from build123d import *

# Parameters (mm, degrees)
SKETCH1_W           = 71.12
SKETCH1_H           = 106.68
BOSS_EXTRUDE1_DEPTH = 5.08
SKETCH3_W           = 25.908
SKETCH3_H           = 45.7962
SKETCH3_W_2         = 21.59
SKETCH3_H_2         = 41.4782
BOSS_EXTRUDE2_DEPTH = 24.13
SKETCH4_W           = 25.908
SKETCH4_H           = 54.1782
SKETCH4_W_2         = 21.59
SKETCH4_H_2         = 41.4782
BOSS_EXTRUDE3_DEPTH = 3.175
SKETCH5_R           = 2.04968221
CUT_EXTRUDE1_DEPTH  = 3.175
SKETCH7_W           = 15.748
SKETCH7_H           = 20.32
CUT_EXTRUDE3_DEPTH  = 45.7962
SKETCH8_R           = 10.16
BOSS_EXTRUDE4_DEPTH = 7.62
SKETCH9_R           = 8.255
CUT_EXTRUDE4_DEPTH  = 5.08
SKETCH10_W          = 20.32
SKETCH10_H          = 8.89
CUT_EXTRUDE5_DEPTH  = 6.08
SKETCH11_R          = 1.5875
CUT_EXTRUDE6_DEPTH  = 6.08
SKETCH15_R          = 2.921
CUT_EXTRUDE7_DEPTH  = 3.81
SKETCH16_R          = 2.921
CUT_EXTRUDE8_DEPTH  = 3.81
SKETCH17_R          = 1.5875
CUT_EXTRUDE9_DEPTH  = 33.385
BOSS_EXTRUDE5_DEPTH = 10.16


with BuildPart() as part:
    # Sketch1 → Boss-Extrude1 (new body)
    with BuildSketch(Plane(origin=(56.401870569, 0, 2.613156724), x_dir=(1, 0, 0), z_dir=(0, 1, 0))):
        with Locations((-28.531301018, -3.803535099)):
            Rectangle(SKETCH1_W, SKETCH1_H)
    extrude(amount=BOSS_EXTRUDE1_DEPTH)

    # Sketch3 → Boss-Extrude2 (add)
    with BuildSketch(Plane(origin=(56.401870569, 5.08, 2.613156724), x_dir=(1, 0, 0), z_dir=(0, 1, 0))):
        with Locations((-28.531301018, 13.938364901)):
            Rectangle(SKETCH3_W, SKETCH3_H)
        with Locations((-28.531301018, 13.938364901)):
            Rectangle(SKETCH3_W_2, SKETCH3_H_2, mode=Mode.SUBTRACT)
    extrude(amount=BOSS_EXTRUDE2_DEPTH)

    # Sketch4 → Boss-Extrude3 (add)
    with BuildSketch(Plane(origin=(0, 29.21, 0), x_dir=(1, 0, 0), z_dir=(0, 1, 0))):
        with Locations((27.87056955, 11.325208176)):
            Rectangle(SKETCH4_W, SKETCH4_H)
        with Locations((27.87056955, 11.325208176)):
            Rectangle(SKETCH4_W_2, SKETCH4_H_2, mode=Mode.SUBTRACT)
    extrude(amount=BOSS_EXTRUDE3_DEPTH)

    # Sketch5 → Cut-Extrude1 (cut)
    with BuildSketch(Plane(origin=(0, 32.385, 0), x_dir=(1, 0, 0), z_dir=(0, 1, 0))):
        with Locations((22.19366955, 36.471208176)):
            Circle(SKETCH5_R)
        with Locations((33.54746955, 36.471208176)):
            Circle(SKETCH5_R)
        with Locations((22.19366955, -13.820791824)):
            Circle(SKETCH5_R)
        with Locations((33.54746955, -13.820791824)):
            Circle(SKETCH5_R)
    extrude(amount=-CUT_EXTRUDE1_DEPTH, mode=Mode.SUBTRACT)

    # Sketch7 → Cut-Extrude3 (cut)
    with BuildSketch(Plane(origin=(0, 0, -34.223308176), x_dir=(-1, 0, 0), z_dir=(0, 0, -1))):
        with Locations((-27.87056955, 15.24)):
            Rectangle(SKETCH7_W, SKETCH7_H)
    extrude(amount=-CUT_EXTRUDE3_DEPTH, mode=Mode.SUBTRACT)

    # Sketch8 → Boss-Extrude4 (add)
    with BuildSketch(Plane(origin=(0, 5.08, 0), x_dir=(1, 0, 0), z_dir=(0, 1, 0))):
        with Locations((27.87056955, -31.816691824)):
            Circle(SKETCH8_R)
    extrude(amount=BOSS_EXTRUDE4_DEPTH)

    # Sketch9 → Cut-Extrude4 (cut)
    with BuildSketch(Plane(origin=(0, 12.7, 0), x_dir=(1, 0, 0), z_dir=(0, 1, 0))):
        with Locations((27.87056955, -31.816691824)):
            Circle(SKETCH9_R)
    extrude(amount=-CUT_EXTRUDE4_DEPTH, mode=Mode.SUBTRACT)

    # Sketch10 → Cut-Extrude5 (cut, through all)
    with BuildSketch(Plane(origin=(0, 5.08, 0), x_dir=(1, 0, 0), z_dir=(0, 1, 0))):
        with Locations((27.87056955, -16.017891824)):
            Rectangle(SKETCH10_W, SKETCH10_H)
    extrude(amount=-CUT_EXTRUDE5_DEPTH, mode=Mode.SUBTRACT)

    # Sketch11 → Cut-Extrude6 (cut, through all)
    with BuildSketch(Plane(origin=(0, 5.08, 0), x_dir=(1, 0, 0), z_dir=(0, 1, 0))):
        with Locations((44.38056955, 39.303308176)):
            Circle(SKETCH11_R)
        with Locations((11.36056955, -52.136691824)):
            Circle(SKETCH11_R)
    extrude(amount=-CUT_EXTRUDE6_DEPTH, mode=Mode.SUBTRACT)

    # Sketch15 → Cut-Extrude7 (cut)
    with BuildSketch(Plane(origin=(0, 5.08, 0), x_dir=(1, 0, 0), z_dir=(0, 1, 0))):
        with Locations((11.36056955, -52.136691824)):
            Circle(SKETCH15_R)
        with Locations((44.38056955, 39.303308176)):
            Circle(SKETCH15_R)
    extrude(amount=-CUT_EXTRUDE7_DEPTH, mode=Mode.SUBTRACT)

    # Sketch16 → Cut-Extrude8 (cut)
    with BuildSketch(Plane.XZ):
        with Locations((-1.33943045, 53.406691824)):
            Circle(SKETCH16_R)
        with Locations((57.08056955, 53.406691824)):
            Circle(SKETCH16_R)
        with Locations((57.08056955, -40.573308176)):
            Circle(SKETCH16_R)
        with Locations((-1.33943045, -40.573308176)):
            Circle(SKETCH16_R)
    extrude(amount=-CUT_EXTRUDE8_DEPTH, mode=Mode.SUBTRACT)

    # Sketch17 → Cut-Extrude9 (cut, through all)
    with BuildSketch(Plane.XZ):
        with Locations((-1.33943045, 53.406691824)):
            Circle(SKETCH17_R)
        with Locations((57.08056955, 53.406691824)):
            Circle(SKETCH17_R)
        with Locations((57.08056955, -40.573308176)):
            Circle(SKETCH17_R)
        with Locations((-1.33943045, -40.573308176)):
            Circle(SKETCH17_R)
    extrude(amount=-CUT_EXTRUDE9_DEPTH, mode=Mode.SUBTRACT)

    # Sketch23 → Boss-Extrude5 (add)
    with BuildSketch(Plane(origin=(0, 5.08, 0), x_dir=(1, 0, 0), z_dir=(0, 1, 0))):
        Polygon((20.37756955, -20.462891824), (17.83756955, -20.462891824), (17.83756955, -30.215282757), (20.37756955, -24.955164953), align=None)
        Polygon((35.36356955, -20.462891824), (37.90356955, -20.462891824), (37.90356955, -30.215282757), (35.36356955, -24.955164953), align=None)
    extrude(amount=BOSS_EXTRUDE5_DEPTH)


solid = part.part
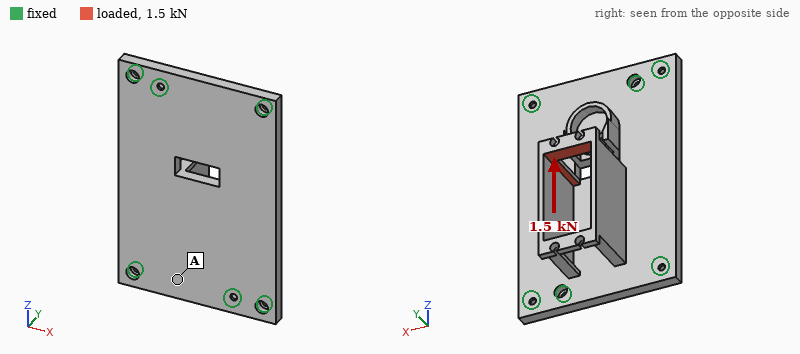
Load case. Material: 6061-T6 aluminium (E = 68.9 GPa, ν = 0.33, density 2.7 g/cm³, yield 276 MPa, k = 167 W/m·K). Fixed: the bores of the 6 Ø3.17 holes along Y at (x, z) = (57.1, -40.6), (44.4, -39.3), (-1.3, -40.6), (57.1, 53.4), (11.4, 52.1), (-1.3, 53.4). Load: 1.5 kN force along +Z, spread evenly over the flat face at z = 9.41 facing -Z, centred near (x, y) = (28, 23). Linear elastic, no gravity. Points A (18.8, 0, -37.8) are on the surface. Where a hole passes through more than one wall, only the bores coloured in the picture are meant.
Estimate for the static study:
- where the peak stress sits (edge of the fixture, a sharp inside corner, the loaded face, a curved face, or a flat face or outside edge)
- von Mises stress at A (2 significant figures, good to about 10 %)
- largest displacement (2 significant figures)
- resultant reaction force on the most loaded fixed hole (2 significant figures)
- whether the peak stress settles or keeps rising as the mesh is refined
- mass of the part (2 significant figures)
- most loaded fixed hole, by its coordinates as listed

a sharp inside corner
16 MPa
0.21 mm
970 N
keeps rising
120 g
(11.4, 52.1)
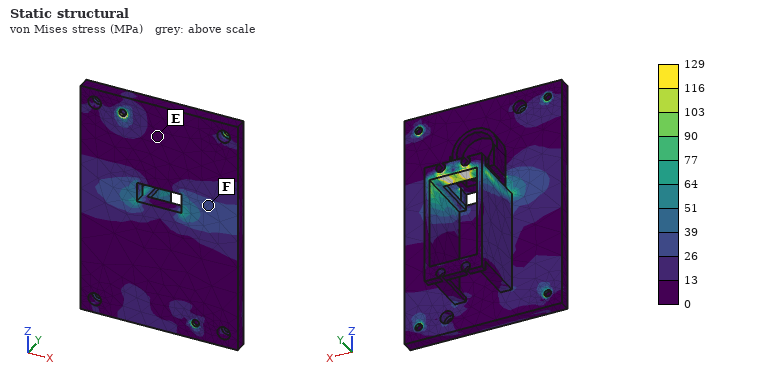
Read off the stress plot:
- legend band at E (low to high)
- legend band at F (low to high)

0 to 13 MPa
26 to 39 MPa
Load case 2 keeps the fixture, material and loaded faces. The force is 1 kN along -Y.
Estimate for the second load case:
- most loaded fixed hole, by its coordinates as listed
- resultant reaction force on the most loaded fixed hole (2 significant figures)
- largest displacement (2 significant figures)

(11.4, 52.1)
1.2 kN
0.20 mm
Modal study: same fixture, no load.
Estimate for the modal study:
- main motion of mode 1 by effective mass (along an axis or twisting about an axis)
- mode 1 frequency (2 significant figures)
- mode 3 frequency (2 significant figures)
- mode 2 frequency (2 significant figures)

along Y
1900 Hz
4600 Hz
2800 Hz
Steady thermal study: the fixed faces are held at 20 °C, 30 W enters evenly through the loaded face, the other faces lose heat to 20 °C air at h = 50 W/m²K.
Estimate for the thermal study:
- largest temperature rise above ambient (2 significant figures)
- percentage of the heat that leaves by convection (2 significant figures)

54 K
37 %
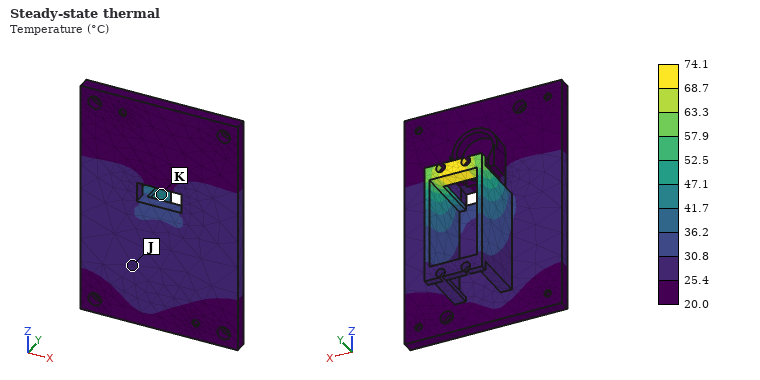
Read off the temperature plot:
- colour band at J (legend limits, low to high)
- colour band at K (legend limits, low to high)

25.4 to 30.8 °C
41.7 to 47.1 °C
